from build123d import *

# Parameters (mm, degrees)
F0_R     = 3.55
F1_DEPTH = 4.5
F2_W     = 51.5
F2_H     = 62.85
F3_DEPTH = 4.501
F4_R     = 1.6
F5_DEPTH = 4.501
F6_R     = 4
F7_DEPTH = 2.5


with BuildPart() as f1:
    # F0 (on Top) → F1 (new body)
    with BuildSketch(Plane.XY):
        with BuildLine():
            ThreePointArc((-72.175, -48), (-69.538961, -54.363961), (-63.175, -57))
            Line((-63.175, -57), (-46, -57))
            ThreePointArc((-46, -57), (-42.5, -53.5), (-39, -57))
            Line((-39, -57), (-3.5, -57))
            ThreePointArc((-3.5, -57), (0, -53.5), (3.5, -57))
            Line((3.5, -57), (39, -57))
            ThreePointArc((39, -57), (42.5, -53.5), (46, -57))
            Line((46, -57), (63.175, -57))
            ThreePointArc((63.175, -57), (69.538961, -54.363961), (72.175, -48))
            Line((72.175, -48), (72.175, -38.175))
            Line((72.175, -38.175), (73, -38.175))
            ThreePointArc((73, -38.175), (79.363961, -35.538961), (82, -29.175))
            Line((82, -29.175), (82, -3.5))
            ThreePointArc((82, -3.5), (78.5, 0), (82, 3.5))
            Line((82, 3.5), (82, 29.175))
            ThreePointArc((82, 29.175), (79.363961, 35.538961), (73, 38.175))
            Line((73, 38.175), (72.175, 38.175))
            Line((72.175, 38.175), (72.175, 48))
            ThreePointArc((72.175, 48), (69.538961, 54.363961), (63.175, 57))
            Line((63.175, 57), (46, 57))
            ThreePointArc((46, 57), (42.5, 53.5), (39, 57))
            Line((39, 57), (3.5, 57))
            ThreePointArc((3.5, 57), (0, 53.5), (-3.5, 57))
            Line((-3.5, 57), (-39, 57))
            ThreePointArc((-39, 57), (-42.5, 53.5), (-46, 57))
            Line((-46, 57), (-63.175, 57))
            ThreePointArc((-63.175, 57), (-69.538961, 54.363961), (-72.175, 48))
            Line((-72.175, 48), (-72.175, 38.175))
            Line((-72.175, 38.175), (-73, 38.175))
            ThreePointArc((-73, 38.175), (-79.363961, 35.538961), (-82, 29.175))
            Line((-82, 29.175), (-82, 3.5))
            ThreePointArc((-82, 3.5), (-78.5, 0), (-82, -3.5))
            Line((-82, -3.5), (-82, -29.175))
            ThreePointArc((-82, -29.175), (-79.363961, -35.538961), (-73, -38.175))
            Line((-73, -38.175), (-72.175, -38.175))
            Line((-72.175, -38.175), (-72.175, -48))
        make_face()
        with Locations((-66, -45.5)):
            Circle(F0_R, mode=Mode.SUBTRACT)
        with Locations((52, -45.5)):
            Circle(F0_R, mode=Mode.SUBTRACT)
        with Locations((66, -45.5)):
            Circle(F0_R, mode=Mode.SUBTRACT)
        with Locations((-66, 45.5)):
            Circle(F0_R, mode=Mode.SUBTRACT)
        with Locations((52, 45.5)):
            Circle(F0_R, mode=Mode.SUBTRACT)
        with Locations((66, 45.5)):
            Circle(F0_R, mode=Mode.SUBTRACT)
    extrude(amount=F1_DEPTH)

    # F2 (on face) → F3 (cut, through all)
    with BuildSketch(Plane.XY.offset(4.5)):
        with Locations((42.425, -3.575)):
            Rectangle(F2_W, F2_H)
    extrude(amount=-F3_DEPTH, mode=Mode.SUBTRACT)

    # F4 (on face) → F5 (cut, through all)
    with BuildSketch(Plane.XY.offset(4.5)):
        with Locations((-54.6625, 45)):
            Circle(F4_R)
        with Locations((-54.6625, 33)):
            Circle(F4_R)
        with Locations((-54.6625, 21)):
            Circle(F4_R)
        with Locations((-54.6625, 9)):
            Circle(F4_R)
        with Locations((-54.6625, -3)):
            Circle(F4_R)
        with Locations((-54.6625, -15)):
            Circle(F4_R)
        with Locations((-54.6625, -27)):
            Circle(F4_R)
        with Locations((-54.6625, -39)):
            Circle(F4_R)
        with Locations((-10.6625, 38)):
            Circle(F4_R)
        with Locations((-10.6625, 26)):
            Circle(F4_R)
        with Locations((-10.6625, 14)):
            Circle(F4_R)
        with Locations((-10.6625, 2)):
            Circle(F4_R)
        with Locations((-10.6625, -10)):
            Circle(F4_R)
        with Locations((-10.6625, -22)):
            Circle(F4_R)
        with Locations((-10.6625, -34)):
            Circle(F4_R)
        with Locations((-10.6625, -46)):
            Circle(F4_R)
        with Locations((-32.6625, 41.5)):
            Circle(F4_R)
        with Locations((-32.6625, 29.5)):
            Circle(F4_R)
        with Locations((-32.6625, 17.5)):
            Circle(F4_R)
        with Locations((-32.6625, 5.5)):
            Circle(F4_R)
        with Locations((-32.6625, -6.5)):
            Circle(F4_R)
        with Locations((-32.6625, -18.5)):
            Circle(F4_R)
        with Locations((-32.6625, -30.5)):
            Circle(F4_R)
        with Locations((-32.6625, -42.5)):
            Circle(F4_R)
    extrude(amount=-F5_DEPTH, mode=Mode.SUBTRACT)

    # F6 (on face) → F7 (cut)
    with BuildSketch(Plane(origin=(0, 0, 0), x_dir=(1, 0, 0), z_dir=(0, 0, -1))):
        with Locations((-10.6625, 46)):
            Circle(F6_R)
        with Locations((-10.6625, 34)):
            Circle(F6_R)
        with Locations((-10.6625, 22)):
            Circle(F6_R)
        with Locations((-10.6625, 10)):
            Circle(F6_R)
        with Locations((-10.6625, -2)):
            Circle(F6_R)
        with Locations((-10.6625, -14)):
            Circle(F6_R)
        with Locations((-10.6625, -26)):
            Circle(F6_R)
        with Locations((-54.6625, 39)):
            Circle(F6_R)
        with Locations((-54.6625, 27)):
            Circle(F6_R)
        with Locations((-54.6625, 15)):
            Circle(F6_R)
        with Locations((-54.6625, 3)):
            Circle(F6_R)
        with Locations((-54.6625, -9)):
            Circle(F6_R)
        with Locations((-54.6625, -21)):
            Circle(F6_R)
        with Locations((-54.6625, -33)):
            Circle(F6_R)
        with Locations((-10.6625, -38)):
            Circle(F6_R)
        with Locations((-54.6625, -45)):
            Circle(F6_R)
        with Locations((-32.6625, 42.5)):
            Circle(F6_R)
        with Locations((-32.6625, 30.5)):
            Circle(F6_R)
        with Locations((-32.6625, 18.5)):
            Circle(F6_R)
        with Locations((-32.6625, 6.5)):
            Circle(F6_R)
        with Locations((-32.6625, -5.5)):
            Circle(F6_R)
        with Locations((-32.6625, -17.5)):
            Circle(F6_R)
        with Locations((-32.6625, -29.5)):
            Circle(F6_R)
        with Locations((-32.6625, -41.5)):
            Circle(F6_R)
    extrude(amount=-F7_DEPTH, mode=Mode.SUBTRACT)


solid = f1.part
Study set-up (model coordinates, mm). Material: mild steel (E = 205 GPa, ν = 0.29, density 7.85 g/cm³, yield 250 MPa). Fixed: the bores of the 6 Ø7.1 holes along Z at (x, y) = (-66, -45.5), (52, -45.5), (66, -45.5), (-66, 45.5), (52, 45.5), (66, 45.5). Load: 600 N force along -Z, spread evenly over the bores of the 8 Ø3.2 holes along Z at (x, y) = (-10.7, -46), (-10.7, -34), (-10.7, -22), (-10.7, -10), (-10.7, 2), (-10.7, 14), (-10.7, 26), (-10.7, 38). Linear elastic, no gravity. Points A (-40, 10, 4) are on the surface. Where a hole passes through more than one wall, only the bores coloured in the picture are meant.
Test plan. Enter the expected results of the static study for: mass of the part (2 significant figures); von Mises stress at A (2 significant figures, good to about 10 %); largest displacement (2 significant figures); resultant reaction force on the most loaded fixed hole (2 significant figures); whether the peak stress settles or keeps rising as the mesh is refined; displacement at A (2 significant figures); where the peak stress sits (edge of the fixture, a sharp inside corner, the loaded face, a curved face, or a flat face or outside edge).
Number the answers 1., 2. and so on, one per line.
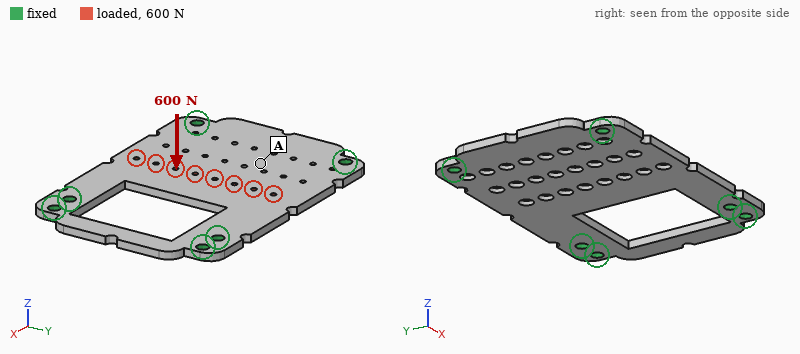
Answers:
1. 470 g
2. 8.4 MPa
3. 64 µm
4. 200 N
5. keeps rising
6. 33 µm
7. edge of the fixture
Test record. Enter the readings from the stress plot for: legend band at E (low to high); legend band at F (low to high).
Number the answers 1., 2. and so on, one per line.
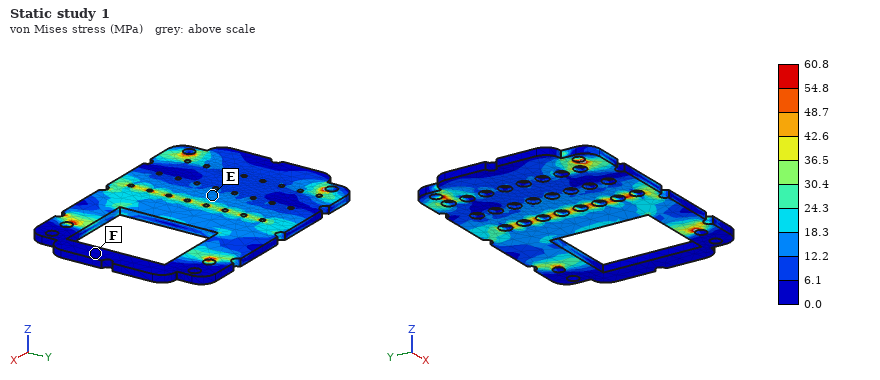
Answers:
1. 12.2 to 18.3 MPa
2. 0.0 to 6.1 MPa
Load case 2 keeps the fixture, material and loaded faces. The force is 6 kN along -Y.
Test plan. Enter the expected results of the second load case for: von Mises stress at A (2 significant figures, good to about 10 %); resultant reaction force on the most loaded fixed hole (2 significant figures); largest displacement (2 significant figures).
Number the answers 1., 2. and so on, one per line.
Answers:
1. 18 MPa
2. 2.9 kN
3. 20 µm
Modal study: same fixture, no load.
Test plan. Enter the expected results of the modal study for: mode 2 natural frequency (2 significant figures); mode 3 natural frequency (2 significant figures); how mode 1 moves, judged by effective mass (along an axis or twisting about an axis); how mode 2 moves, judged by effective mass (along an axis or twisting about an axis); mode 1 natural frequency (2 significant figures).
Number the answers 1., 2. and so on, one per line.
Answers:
1. 1900 Hz
2. 2600 Hz
3. along Z
4. twisting about X
5. 1300 Hz
